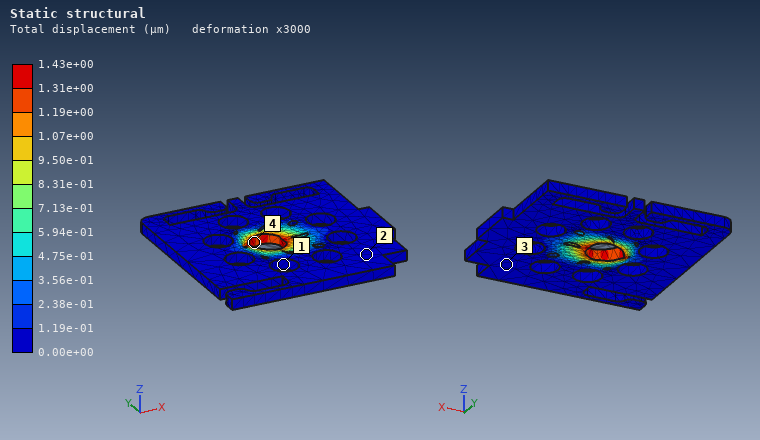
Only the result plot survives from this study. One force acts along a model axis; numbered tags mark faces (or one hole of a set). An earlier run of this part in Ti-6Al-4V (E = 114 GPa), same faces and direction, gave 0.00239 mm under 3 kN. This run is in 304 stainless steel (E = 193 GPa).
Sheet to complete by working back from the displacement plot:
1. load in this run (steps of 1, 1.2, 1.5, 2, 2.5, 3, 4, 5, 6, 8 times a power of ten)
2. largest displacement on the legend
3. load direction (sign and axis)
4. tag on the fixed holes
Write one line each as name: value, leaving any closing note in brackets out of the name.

load in this run: 3 kN
largest displacement on the legend: 1.43e+00 µm
load direction: -X
tag on the fixed holes: 1
